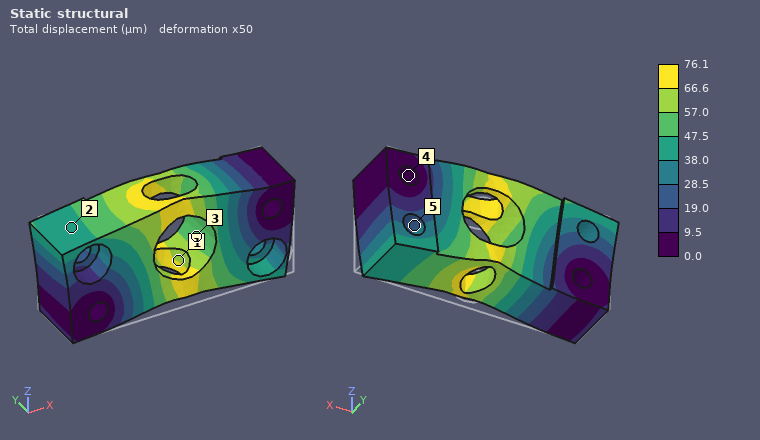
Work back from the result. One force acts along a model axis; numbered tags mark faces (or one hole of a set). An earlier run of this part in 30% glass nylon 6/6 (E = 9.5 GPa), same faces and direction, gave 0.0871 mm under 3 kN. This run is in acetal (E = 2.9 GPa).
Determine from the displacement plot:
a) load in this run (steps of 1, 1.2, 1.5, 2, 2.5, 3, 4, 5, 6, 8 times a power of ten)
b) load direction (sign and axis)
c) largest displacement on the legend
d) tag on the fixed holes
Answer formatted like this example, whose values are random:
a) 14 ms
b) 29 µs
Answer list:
a) 800 N
b) +Z
c) 76.1 µm
d) 4
